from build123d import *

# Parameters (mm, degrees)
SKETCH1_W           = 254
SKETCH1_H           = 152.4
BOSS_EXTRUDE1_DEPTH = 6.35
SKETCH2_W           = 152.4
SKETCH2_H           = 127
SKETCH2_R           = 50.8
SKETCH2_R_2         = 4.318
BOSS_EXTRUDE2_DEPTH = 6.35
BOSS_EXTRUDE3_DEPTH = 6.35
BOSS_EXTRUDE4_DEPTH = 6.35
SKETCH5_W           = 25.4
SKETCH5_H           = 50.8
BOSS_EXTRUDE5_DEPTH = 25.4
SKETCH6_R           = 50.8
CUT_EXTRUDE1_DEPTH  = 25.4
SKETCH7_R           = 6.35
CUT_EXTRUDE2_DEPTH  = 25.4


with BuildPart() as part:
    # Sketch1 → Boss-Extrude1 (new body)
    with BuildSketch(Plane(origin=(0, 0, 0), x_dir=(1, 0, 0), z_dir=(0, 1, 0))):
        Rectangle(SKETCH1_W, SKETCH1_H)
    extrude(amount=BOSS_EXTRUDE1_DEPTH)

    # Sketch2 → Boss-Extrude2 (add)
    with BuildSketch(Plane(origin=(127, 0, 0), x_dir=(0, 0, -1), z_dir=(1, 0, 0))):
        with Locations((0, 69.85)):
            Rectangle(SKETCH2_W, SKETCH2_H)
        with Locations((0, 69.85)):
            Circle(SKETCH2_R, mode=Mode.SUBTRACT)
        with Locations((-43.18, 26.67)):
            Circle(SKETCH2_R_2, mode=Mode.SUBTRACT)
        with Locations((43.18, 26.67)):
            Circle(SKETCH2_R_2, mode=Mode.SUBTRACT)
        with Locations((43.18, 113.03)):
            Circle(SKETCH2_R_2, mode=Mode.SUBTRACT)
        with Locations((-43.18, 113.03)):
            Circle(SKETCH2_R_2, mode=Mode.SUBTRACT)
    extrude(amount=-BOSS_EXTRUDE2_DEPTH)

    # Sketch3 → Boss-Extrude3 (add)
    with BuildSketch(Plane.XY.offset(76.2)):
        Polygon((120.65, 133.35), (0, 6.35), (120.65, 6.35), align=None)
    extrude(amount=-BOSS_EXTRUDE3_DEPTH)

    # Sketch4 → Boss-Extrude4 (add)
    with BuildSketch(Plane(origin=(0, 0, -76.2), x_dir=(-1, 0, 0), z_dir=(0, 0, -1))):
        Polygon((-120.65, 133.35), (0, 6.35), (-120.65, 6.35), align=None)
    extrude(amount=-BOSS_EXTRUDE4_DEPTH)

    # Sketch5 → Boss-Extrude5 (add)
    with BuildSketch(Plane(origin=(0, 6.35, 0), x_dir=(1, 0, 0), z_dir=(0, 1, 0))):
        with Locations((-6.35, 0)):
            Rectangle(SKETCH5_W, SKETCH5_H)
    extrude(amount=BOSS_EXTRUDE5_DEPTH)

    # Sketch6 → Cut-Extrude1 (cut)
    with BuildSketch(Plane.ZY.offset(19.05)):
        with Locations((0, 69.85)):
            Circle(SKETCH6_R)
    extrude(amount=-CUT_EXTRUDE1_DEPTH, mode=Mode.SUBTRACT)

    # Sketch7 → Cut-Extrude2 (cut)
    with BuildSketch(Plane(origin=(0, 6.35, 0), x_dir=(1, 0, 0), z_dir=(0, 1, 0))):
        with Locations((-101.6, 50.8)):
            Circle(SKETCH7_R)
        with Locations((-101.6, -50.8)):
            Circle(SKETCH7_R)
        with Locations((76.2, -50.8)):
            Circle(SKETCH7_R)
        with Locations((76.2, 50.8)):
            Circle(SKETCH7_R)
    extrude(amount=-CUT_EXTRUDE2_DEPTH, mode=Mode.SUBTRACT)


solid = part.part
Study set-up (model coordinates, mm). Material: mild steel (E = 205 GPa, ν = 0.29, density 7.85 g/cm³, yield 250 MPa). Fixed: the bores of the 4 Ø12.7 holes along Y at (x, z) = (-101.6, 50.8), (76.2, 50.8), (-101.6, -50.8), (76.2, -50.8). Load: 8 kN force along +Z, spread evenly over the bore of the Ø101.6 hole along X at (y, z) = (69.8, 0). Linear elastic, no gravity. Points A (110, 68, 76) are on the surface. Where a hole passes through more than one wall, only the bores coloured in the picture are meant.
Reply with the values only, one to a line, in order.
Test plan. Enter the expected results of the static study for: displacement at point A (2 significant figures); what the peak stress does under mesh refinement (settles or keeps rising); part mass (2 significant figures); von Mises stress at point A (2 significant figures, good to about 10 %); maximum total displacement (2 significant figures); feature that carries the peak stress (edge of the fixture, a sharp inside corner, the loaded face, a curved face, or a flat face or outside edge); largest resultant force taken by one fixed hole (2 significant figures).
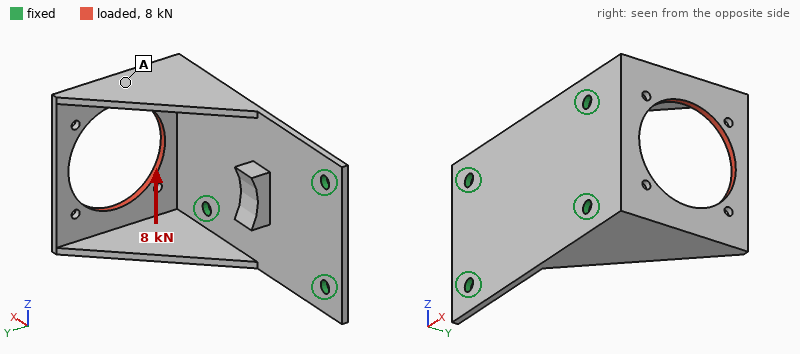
0.26 mm
keeps rising
3.4 kg
22 MPa
0.49 mm
edge of the fixture
7.1 kN
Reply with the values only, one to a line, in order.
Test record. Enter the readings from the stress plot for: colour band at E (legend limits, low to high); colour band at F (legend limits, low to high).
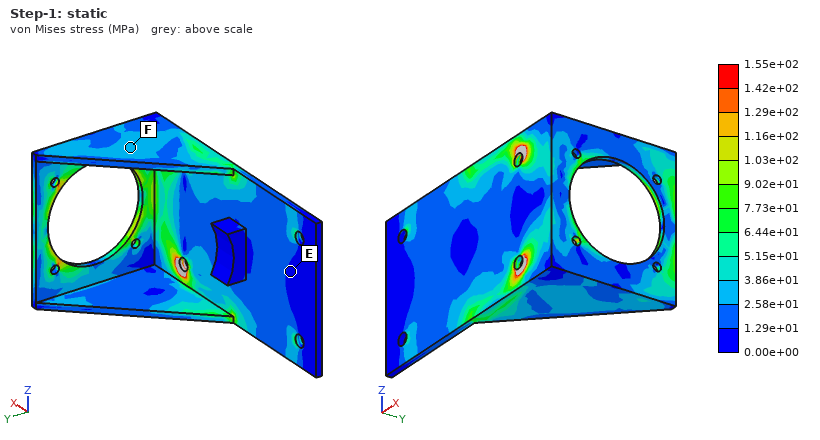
0.00e+00 to 1.29e+01 MPa
2.58e+01 to 3.86e+01 MPa
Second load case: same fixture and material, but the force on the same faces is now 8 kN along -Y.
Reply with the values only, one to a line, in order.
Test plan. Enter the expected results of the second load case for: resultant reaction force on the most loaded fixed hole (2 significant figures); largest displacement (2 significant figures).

4.7 kN
0.38 mm
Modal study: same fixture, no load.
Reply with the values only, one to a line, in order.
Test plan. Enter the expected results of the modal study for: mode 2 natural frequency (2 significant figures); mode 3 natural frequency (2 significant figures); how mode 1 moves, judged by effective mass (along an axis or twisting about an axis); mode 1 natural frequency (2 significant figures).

630 Hz
1200 Hz
along X
590 Hz
